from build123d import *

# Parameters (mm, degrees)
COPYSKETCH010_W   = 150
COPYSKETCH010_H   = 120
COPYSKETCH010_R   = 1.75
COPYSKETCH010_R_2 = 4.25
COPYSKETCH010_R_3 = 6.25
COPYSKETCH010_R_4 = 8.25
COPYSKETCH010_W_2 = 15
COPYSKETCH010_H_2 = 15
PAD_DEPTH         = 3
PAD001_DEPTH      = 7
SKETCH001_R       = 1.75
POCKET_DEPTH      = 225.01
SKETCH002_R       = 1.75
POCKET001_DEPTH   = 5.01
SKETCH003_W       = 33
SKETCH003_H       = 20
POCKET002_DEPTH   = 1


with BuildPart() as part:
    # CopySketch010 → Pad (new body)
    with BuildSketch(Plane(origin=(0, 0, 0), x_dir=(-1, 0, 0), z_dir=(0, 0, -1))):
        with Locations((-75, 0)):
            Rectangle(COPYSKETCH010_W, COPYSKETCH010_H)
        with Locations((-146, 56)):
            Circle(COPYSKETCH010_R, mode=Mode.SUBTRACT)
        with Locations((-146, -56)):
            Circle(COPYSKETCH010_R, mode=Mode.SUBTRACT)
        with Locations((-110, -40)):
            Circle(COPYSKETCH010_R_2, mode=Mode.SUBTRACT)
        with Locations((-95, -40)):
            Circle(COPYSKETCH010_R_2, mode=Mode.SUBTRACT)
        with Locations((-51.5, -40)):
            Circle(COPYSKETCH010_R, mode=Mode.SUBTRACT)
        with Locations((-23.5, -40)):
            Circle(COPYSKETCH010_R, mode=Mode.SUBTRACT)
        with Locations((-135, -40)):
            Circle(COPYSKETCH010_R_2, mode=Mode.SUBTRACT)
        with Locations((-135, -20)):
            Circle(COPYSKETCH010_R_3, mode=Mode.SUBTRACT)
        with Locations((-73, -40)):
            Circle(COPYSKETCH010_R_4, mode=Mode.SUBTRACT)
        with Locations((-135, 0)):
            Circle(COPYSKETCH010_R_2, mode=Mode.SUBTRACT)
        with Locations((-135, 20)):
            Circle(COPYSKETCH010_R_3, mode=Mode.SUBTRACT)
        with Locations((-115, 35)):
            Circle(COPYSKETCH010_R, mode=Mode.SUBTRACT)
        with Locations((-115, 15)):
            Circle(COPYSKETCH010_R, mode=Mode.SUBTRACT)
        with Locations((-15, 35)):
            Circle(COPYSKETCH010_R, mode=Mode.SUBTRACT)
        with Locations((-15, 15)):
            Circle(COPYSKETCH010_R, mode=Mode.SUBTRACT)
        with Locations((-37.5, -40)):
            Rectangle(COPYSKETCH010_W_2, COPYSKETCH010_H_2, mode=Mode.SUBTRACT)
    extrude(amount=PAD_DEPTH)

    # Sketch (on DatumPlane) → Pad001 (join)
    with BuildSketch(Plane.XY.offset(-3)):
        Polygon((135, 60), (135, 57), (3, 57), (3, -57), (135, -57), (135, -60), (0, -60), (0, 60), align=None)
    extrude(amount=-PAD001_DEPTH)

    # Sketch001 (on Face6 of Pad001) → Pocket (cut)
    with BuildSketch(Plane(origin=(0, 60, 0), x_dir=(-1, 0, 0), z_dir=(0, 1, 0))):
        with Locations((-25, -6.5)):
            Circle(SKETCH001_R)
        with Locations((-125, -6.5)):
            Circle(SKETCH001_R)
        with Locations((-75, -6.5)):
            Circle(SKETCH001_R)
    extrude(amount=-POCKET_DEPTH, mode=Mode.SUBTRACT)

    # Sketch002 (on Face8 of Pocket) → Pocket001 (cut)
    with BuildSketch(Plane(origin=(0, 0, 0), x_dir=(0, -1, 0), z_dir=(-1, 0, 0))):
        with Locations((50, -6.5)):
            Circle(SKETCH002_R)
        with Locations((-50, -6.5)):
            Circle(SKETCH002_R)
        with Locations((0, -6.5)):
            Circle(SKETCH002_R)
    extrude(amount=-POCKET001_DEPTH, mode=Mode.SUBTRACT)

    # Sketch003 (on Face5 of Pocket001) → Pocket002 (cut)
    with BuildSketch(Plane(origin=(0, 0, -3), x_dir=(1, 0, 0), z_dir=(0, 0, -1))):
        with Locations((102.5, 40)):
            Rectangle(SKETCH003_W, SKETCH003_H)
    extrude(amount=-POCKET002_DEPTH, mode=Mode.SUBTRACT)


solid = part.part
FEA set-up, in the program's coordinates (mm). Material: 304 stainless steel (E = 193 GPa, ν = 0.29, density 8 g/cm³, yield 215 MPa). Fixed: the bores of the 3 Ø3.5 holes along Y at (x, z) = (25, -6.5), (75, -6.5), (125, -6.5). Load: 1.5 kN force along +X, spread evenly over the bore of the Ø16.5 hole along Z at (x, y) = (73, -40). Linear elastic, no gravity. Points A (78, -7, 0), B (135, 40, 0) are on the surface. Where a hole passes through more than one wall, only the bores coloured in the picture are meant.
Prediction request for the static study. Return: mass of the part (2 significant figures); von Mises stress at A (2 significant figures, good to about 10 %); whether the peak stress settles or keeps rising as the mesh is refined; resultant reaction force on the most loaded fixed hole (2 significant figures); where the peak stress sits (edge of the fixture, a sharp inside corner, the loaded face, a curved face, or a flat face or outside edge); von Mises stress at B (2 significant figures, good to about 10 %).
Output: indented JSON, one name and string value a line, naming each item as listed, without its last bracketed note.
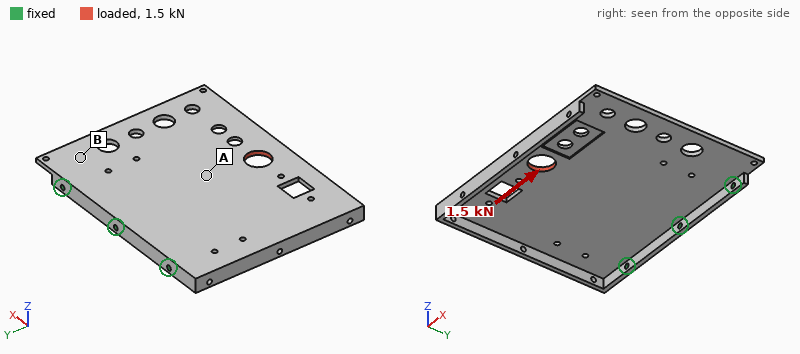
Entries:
{
  "mass of the part": "470 g",
  "von Mises stress at A": "6.7 MPa",
  "whether the peak stress settles or keeps rising as the mesh is refined": "keeps rising",
  "resultant reaction force on the most loaded fixed hole": "1.5 kN",
  "where the peak stress sits": "edge of the fixture",
  "von Mises stress at B": "11 MPa"
}
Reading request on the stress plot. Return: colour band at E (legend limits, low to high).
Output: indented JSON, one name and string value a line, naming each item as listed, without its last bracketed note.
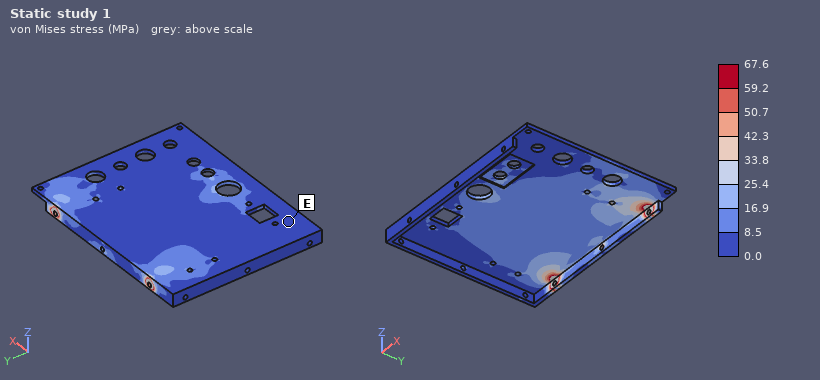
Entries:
{
  "colour band at E": "0.0 to 8.5 MPa"
}
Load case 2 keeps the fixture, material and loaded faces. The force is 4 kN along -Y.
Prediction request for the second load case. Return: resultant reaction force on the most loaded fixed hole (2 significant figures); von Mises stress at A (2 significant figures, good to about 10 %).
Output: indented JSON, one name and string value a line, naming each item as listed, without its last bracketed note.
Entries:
{
  "resultant reaction force on the most loaded fixed hole": "1.4 kN",
  "von Mises stress at A": "21 MPa"
}
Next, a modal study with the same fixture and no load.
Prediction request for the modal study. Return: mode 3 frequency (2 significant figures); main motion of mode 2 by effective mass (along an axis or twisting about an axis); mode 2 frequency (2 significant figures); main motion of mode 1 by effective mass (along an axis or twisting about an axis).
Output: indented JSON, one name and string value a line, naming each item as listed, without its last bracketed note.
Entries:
{
  "mode 3 frequency": "930 Hz",
  "main motion of mode 2 by effective mass": "twisting about Y",
  "mode 2 frequency": "310 Hz",
  "main motion of mode 1 by effective mass": "along Z"
}
